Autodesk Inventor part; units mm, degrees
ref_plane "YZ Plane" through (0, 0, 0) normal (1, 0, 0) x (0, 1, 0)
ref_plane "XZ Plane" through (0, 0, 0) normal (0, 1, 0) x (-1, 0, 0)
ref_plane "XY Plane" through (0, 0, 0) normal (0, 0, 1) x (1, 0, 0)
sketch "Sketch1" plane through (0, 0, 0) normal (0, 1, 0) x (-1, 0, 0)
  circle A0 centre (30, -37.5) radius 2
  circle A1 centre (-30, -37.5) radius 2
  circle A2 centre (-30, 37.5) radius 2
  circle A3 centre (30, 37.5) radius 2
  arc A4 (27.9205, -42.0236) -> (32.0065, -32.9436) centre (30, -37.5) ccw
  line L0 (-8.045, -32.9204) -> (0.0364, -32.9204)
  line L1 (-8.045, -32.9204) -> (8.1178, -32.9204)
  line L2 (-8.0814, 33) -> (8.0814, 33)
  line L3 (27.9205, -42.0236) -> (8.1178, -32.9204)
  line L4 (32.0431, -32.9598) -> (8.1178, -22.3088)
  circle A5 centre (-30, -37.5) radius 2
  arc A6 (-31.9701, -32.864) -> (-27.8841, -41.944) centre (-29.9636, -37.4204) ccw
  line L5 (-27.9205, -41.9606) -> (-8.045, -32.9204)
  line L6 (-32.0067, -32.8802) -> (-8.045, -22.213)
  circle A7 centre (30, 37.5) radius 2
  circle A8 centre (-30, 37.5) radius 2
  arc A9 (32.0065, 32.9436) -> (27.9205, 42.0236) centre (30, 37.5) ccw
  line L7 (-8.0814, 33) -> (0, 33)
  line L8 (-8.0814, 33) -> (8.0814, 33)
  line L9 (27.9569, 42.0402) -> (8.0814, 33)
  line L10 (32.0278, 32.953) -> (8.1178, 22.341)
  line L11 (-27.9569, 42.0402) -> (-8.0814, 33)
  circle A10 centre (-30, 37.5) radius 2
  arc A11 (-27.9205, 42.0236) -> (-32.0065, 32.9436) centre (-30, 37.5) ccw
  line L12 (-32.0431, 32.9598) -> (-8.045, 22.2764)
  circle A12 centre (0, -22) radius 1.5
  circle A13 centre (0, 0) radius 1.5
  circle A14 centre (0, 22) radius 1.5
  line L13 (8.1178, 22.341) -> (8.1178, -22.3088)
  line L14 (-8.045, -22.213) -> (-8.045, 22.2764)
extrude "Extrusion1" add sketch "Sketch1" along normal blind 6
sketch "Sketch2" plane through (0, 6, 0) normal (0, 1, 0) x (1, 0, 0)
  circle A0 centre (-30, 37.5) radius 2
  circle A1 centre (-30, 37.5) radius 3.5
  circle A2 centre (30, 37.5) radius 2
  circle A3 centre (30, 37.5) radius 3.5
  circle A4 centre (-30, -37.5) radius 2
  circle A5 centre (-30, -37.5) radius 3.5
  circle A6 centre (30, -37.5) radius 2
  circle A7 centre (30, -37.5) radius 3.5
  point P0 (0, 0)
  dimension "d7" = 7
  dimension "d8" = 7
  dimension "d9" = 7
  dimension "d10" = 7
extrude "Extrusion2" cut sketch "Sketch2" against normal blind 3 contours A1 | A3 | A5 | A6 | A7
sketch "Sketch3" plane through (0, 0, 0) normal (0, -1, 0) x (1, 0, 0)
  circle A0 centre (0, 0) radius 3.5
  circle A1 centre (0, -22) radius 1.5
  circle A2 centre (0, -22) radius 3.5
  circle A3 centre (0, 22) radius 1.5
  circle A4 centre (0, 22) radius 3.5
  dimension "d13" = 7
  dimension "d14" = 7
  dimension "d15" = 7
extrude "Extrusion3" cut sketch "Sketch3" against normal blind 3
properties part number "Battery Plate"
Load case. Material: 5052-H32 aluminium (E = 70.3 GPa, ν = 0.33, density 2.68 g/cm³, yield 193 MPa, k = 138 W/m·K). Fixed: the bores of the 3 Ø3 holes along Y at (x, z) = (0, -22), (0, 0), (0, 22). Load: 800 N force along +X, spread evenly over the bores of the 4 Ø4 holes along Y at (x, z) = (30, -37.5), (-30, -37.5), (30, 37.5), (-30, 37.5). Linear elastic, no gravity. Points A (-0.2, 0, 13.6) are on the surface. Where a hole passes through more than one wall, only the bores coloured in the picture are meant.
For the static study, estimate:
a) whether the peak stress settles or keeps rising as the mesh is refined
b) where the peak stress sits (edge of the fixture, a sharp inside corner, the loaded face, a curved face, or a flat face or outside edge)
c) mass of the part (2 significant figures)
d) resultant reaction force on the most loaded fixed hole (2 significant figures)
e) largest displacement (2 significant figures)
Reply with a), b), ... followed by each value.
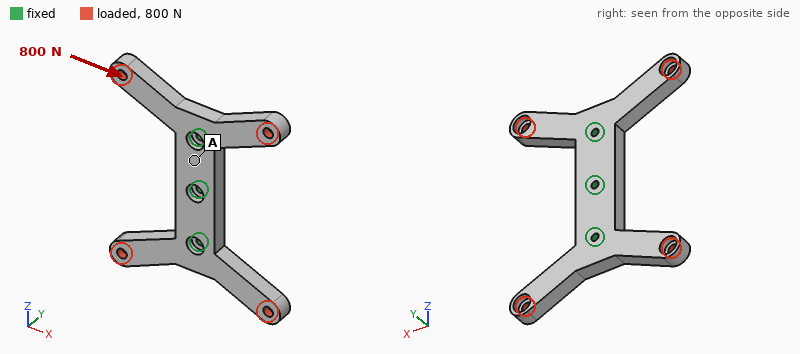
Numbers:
a) keeps rising
b) edge of the fixture
c) 32 g
d) 610 N
e) 67 µm
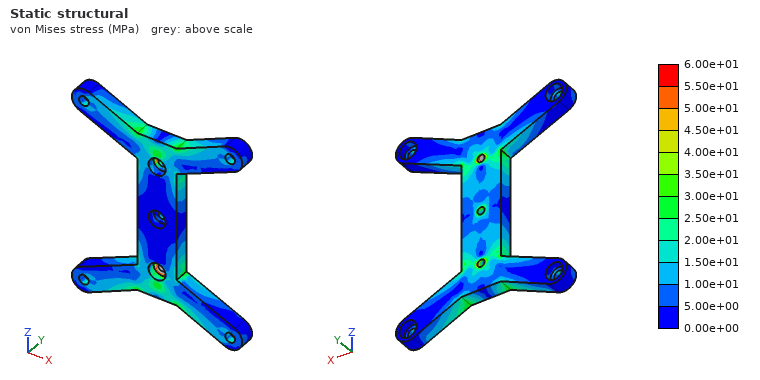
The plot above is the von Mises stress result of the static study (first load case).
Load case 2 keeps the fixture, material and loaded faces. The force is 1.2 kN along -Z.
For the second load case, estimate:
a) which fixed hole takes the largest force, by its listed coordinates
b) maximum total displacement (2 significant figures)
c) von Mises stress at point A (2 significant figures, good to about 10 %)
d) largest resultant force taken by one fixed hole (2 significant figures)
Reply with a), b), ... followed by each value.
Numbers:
a) (0, 0)
b) 92 µm
c) 7.5 MPa
d) 570 N
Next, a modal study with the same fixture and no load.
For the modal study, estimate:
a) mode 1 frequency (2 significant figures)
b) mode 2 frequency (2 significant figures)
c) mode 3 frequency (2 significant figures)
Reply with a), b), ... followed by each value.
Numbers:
a) 2700 Hz
b) 2800 Hz
c) 4100 Hz
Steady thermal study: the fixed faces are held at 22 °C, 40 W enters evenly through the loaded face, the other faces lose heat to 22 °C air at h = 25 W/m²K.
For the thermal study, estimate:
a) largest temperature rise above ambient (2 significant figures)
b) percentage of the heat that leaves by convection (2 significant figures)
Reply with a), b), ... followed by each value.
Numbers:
a) 49 K
b) 8.9 %
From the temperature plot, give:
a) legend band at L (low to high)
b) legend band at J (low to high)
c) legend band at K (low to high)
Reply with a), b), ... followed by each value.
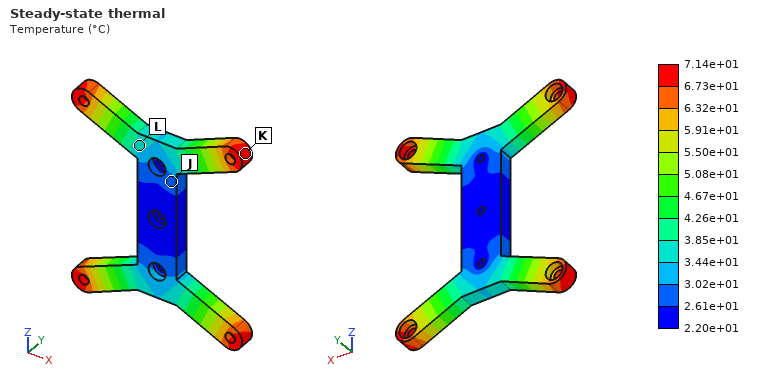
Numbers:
a) 3.44e+01 to 3.85e+01 °C
b) 2.61e+01 to 3.02e+01 °C
c) 6.73e+01 to 7.14e+01 °C
